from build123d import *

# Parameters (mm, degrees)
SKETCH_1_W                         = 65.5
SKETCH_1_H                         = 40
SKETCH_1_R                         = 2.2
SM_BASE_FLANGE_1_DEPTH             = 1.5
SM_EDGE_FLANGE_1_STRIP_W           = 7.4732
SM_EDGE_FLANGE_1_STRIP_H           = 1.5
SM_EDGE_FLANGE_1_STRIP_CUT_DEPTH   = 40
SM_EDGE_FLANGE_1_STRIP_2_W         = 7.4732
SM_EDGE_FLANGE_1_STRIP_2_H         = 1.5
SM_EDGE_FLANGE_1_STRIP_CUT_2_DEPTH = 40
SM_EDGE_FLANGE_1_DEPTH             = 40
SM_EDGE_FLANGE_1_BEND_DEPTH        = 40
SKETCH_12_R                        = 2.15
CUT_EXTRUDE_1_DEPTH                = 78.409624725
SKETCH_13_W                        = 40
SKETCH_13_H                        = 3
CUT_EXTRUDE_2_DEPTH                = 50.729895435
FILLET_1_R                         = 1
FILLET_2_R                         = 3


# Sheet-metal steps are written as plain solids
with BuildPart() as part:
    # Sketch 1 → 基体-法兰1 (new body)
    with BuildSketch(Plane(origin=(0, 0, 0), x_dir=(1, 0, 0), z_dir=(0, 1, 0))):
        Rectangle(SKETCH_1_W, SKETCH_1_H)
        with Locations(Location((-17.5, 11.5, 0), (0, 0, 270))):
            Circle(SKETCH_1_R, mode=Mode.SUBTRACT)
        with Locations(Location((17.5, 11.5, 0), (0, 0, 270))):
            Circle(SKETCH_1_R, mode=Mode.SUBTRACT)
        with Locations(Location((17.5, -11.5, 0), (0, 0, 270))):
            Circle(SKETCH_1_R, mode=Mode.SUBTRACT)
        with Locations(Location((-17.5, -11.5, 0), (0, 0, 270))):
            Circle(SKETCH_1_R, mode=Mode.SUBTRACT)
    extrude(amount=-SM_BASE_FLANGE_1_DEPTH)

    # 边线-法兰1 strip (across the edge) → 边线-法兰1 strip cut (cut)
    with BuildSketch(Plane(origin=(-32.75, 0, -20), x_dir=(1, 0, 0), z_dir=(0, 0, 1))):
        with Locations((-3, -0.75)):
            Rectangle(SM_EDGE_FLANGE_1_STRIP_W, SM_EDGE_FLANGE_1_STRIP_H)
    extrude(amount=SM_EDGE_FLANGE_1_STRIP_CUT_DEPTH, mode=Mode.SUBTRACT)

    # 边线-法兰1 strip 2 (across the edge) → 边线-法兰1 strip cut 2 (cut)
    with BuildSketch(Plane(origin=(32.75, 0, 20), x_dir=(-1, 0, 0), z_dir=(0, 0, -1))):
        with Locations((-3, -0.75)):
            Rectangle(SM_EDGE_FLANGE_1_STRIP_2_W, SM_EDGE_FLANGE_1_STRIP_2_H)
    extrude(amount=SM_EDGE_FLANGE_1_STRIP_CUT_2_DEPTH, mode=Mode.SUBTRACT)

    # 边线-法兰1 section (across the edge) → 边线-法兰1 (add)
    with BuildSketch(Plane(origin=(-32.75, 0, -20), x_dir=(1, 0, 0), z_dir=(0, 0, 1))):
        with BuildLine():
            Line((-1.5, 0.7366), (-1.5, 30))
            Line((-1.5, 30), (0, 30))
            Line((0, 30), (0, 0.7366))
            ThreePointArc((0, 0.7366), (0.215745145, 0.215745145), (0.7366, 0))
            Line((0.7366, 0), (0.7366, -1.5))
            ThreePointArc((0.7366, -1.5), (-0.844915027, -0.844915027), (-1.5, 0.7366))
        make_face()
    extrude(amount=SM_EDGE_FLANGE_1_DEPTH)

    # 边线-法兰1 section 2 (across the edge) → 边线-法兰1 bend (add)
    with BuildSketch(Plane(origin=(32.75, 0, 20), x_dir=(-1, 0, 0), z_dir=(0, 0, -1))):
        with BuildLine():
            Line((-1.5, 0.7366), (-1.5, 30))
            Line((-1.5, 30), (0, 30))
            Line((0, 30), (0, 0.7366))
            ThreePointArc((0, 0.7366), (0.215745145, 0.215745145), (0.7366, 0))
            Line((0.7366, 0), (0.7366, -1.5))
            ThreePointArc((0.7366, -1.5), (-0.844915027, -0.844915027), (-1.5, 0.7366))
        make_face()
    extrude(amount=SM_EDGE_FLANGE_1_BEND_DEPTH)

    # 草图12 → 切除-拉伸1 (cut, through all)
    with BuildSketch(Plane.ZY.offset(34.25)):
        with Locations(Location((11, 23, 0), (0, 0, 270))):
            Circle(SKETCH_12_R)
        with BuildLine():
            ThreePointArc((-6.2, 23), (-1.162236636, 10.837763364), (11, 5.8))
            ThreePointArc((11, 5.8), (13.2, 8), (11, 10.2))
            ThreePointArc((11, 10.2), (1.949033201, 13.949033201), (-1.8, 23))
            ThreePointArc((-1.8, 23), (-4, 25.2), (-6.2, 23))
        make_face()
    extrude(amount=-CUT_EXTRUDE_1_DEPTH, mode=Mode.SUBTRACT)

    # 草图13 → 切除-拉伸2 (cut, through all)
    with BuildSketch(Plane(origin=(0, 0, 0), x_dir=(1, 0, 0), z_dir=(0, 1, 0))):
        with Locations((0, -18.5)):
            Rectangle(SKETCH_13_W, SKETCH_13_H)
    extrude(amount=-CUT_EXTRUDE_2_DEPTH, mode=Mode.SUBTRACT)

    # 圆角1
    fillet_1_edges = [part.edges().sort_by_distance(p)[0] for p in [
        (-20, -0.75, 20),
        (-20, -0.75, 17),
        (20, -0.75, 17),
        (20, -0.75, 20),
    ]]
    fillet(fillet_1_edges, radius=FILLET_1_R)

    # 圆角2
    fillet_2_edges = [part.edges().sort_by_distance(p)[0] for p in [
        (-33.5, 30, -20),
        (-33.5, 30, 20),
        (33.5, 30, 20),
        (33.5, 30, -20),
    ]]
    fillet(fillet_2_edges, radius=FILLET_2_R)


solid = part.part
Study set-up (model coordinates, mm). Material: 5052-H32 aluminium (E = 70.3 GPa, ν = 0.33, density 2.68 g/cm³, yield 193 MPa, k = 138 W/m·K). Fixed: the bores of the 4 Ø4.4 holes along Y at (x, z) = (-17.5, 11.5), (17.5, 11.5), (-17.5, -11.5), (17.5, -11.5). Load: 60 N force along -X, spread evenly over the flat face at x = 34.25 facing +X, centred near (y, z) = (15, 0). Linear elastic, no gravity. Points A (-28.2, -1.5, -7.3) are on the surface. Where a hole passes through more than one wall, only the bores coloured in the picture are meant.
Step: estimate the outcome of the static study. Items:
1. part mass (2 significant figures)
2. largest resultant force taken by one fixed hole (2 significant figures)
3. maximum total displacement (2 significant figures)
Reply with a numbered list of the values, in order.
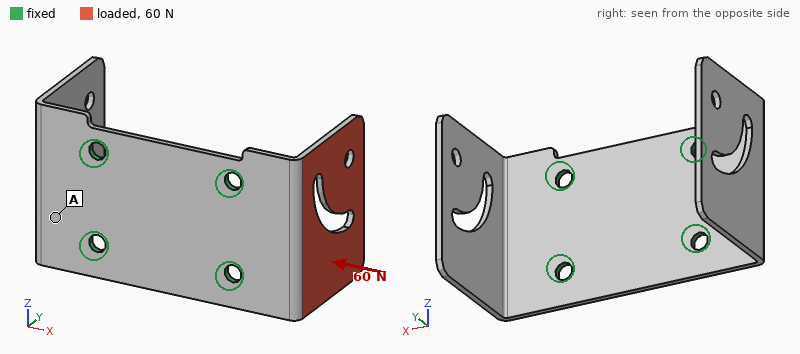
1. 19 g
2. 28 N
3. 0.93 mm
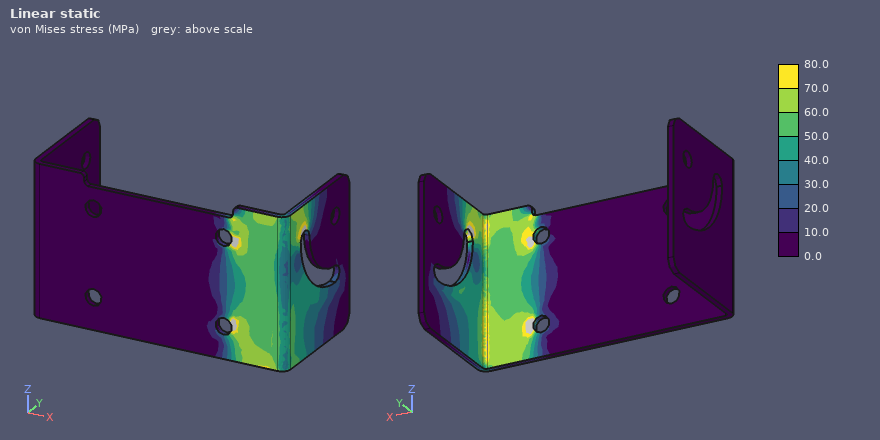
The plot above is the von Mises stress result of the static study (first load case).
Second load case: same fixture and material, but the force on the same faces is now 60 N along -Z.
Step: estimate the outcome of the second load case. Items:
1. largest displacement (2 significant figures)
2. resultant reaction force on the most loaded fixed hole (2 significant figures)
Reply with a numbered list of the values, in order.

1. 0.15 mm
2. 59 N
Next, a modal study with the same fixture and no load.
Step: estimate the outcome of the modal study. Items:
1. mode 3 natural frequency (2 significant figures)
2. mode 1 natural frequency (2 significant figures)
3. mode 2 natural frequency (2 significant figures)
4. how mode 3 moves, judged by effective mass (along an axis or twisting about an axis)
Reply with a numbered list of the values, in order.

1. 1600 Hz
2. 750 Hz
3. 760 Hz
4. along Z
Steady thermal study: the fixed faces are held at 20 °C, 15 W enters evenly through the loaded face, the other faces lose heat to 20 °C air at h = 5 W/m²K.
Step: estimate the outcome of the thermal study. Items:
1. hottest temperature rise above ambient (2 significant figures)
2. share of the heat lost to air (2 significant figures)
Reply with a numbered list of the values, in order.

1. 78 K
2. 3.4 %
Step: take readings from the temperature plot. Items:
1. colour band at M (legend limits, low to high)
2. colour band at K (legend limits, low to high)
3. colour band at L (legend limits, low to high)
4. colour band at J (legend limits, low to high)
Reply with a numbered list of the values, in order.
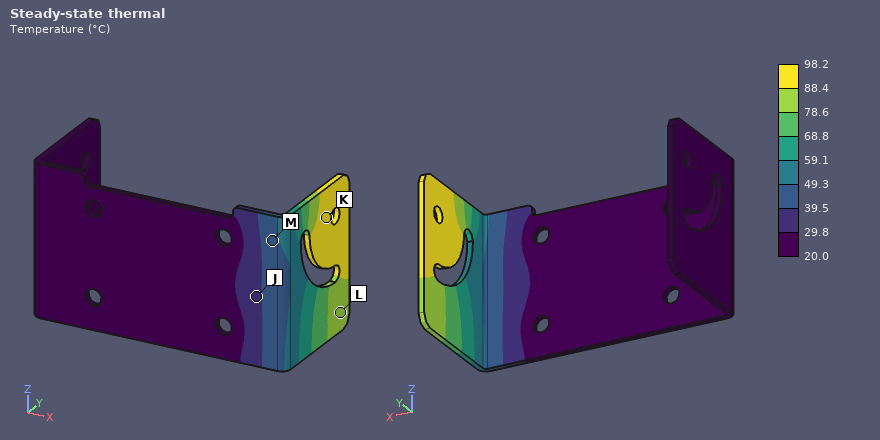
1. 39.5 to 49.3 °C
2. 88.4 to 98.2 °C
3. 78.6 to 88.4 °C
4. 29.8 to 39.5 °C
